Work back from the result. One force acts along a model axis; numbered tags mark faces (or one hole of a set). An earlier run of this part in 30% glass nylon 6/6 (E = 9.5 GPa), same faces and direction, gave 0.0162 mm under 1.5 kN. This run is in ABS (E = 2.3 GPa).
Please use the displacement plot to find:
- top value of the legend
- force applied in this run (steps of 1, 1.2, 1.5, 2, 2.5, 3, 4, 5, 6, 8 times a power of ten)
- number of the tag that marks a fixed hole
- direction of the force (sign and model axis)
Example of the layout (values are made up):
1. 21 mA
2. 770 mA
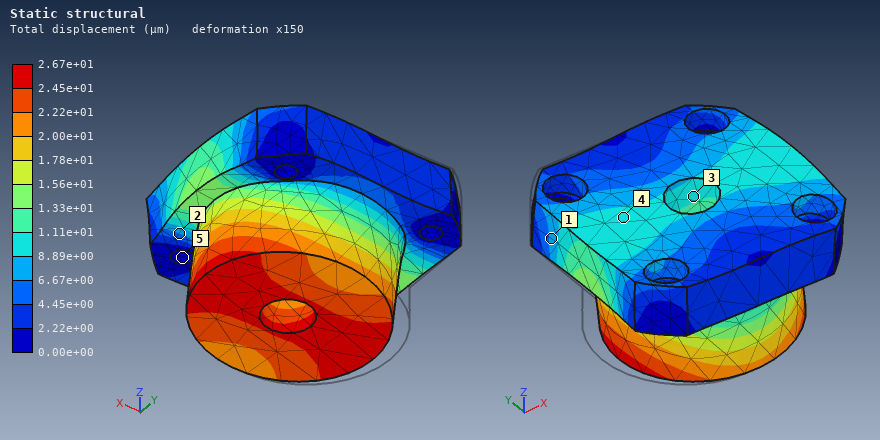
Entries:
1. 2.67e+01 µm
2. 600 N
3. 5
4. +X
